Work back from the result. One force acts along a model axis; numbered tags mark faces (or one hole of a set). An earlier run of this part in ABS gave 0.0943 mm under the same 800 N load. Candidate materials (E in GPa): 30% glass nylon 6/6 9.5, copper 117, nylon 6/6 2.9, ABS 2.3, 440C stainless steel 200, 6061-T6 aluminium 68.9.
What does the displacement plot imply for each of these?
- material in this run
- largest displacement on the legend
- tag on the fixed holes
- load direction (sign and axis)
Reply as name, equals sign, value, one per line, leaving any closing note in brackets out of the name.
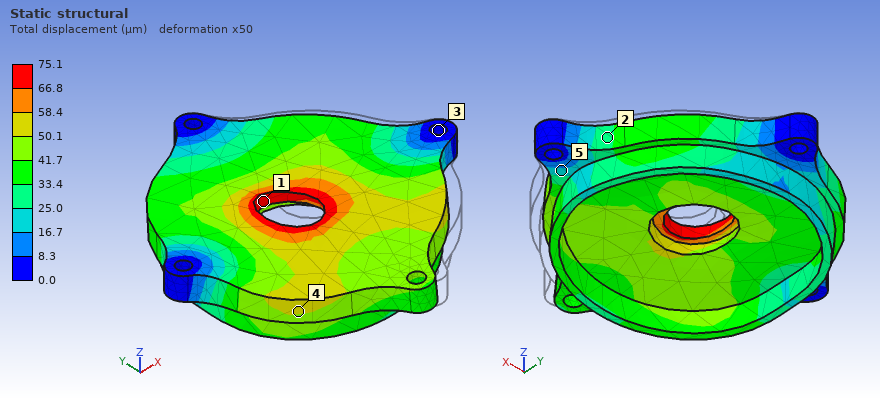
material in this run = nylon 6/6
largest displacement on the legend = 75.1 µm
tag on the fixed holes = 3
load direction = -X
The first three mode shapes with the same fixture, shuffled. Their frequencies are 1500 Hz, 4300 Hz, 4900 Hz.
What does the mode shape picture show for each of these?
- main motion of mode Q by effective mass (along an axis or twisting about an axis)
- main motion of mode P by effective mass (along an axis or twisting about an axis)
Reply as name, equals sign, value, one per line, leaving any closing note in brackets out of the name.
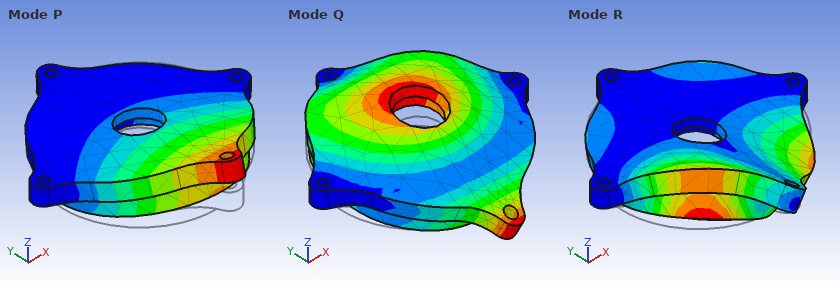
main motion of mode Q by effective mass = along Z
main motion of mode P by effective mass = along Z
